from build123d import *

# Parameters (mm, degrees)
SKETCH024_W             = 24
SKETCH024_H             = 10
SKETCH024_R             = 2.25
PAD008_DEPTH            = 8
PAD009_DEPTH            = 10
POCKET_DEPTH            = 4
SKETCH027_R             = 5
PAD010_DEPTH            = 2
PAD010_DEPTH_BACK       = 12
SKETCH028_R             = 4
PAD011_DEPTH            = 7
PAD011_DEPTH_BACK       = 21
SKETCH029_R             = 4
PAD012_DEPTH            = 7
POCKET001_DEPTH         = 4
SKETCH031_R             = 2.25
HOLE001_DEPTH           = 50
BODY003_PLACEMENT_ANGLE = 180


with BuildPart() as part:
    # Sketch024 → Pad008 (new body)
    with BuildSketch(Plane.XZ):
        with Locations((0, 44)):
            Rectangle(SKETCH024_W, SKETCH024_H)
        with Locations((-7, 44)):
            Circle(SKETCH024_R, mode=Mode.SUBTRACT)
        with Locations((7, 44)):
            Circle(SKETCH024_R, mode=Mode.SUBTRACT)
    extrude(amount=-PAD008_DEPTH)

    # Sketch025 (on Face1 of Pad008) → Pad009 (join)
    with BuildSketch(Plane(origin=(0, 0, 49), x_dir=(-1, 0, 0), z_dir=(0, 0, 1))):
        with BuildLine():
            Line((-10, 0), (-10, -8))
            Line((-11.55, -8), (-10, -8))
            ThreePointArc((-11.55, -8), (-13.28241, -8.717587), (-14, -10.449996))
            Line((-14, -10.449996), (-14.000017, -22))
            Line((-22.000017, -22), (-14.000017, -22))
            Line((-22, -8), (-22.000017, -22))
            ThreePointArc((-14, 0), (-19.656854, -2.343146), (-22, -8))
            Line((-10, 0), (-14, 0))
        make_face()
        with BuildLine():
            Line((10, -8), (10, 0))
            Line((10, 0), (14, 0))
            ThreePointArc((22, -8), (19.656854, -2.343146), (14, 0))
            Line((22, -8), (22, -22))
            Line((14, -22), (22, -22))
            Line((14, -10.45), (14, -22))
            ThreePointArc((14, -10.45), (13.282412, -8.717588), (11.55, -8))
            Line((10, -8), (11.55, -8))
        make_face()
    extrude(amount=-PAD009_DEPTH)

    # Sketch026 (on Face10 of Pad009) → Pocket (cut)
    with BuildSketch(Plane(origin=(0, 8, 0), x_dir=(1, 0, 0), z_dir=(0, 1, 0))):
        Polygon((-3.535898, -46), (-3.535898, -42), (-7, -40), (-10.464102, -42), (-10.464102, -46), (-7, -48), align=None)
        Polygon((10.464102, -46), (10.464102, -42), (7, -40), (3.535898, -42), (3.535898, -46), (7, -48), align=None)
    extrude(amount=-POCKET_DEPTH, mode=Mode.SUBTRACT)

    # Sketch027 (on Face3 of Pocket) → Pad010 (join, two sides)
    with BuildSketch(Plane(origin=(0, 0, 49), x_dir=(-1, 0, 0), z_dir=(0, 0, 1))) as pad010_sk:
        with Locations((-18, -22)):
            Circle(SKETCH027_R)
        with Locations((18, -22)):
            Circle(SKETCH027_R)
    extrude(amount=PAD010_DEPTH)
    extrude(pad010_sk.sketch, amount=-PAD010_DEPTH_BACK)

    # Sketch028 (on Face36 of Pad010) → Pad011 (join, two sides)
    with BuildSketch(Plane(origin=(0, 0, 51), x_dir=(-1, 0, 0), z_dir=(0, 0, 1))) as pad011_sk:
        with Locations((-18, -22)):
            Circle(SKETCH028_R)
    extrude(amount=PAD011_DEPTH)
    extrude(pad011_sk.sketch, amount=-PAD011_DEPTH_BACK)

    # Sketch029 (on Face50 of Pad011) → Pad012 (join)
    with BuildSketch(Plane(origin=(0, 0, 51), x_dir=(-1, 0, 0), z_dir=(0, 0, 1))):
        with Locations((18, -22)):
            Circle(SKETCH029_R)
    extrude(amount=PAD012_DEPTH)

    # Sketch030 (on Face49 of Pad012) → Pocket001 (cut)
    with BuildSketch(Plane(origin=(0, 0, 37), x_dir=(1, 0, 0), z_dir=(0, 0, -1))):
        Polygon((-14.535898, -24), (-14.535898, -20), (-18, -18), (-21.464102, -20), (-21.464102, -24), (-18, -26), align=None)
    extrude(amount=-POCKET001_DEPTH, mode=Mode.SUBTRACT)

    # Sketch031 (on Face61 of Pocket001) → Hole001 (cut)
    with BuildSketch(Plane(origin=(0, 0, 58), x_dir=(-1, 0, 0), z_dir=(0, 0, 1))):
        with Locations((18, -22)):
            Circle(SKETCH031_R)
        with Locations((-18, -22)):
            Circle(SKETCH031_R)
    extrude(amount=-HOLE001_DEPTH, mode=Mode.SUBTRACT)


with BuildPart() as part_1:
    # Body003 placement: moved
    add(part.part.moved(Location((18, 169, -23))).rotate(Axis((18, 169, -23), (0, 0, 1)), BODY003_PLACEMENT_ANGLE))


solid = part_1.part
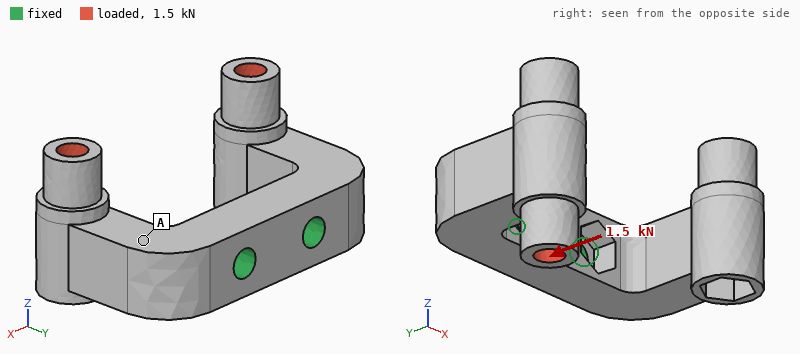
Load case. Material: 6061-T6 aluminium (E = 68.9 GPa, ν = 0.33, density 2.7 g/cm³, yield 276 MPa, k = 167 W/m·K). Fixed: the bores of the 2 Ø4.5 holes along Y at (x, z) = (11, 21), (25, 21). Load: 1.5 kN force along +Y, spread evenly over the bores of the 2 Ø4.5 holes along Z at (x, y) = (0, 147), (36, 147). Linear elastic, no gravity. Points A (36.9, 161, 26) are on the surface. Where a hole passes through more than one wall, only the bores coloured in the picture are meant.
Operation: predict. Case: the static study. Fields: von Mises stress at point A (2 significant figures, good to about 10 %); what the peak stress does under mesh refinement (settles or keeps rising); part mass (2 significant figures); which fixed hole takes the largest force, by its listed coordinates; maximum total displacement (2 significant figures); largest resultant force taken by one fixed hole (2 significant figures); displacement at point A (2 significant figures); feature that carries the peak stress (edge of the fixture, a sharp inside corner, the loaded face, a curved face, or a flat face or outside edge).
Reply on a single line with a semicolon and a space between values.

27 MPa; keeps rising; 18 g; (11, 21); 0.10 mm; 1.2 kN; 0.036 mm; edge of the fixture
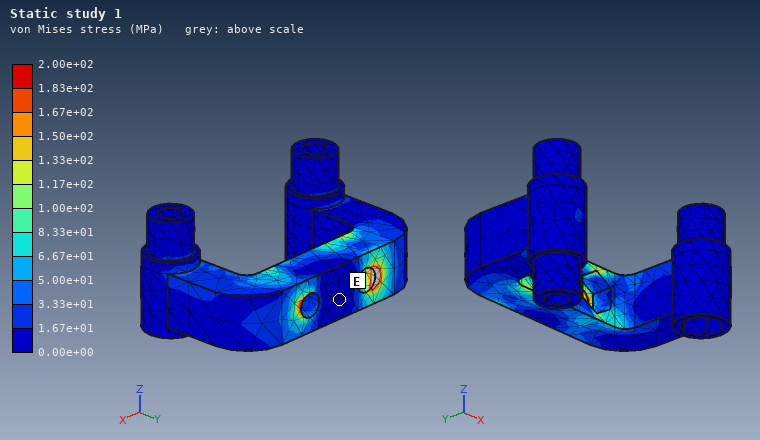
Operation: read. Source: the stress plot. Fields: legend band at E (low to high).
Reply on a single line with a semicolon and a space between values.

0.00e+00 to 1.67e+01 MPa
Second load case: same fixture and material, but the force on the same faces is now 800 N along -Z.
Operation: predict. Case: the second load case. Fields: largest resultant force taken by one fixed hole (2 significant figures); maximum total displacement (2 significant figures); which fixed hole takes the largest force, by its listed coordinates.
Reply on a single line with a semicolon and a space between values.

530 N; 0.18 mm; (11, 21)
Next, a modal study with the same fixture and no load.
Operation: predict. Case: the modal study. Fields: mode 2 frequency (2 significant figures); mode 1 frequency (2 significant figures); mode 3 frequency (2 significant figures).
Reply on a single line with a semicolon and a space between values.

4500 Hz; 4500 Hz; 4900 Hz
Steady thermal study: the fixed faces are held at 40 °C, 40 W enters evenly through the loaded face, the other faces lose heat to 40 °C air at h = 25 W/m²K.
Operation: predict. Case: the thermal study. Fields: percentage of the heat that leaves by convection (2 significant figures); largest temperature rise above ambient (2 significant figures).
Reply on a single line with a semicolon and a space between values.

5.7 %; 51 K
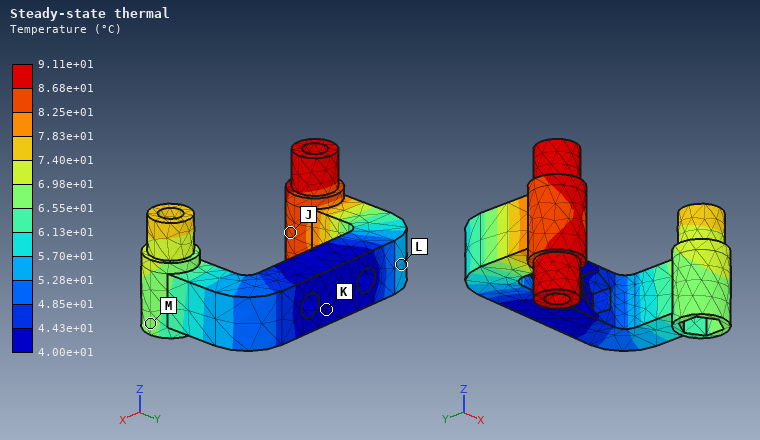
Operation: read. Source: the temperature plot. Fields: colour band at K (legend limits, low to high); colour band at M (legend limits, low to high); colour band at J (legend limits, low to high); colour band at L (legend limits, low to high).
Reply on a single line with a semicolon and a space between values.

4.00e+01 to 4.43e+01 °C; 6.55e+01 to 6.98e+01 °C; 8.25e+01 to 8.68e+01 °C; 5.28e+01 to 5.70e+01 °C
